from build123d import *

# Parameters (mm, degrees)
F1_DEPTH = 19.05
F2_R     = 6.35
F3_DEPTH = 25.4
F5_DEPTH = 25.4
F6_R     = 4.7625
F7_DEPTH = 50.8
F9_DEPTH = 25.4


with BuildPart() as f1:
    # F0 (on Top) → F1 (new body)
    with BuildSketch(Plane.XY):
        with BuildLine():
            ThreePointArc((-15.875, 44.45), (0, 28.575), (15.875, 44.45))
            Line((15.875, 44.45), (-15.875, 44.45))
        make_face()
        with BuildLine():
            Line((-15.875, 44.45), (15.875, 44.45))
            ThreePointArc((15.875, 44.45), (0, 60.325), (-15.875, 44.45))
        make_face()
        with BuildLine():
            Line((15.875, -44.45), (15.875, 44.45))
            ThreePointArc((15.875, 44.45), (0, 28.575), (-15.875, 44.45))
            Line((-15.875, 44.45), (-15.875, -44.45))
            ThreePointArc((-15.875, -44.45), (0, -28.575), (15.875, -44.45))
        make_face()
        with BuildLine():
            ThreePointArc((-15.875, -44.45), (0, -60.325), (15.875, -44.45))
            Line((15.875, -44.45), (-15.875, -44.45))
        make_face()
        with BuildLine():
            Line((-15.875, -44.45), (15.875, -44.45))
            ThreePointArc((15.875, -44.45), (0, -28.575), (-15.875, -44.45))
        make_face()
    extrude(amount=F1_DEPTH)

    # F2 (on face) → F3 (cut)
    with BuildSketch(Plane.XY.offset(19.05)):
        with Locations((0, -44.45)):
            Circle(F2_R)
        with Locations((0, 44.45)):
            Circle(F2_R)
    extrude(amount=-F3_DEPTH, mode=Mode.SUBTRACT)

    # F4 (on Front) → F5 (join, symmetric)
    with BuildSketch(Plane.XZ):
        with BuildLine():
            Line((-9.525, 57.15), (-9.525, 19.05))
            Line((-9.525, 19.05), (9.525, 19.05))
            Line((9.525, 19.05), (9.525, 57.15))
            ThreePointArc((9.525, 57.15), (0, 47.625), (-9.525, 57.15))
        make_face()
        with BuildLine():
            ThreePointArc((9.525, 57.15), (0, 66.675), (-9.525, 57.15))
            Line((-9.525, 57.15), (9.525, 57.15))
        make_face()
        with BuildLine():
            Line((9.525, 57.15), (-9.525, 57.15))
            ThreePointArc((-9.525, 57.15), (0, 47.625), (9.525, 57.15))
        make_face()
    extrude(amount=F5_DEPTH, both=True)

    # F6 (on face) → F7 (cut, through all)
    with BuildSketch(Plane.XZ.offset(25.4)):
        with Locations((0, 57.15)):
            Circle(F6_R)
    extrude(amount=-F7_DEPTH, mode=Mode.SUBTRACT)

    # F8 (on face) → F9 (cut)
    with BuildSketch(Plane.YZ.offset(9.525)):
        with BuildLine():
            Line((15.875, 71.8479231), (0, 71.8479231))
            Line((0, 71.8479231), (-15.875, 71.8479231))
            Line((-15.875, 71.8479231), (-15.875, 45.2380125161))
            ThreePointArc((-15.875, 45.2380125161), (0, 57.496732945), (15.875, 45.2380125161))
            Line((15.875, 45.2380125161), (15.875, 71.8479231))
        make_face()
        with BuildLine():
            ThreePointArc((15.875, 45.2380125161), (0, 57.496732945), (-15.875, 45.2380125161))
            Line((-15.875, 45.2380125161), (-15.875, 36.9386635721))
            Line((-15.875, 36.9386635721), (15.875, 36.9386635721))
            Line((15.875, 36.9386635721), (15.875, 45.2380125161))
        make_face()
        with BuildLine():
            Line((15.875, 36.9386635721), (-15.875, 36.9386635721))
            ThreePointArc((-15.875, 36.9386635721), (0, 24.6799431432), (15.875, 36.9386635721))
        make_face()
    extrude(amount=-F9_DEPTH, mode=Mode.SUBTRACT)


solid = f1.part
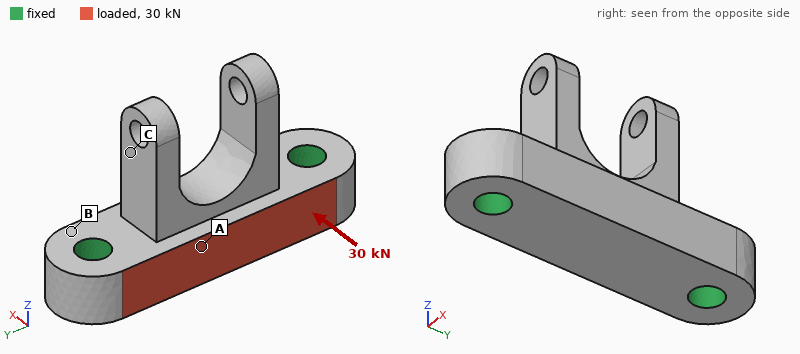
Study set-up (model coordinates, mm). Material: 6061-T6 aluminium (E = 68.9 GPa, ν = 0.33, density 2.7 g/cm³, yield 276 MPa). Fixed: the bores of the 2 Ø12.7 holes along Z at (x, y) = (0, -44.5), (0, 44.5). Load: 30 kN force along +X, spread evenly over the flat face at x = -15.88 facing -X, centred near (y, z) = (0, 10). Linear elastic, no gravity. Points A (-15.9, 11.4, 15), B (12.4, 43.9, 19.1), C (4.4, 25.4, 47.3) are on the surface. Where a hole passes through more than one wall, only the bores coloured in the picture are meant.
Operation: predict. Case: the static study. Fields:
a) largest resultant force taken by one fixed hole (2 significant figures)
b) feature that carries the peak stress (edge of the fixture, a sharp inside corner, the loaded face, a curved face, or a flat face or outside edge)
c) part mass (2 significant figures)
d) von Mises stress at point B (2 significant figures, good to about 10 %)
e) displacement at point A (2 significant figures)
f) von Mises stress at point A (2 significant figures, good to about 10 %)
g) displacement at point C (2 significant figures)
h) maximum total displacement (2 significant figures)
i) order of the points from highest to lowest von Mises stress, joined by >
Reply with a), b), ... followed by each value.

a) 15 kN
b) edge of the fixture
c) 230 g
d) 22 MPa
e) 38 µm
f) 38 MPa
g) 31 µm
h) 44 µm
i) A > B > C
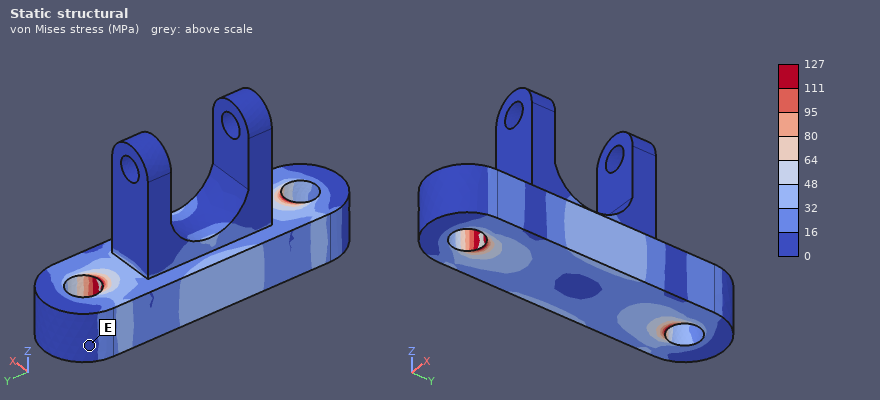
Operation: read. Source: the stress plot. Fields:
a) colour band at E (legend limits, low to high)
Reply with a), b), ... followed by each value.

a) 0 to 16 MPa
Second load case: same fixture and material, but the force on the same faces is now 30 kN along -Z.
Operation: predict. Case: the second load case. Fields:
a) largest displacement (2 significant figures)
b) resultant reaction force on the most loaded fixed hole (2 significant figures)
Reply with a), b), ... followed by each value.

a) 0.18 mm
b) 15 kN
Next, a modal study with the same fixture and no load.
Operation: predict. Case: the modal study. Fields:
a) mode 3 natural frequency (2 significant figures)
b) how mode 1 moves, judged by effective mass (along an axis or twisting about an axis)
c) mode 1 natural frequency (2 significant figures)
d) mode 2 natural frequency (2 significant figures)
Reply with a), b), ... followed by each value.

a) 5800 Hz
b) along X
c) 5200 Hz
d) 5700 Hz
